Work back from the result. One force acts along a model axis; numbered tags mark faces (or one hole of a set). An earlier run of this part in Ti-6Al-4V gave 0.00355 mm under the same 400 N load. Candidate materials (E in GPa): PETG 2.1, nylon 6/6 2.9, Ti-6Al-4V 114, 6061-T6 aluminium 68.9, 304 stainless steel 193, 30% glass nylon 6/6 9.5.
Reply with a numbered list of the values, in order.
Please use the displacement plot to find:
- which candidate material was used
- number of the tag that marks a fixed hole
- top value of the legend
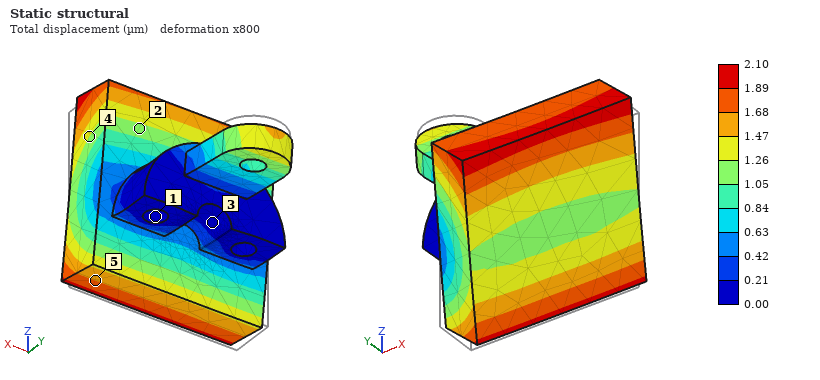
1. 304 stainless steel
2. 1
3. 2.10 µm
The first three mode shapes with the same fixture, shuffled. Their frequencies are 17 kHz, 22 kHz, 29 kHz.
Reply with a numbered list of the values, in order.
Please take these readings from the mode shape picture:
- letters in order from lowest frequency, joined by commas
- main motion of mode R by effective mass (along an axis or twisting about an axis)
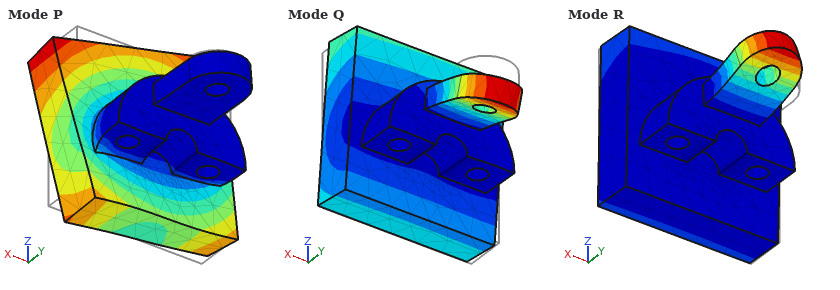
1. Q, R, P
2. along Z
